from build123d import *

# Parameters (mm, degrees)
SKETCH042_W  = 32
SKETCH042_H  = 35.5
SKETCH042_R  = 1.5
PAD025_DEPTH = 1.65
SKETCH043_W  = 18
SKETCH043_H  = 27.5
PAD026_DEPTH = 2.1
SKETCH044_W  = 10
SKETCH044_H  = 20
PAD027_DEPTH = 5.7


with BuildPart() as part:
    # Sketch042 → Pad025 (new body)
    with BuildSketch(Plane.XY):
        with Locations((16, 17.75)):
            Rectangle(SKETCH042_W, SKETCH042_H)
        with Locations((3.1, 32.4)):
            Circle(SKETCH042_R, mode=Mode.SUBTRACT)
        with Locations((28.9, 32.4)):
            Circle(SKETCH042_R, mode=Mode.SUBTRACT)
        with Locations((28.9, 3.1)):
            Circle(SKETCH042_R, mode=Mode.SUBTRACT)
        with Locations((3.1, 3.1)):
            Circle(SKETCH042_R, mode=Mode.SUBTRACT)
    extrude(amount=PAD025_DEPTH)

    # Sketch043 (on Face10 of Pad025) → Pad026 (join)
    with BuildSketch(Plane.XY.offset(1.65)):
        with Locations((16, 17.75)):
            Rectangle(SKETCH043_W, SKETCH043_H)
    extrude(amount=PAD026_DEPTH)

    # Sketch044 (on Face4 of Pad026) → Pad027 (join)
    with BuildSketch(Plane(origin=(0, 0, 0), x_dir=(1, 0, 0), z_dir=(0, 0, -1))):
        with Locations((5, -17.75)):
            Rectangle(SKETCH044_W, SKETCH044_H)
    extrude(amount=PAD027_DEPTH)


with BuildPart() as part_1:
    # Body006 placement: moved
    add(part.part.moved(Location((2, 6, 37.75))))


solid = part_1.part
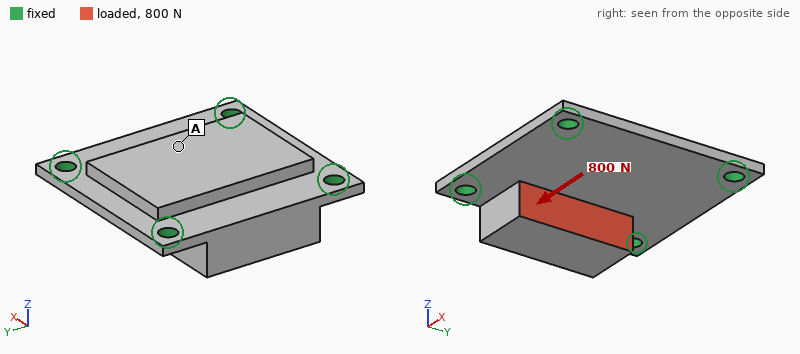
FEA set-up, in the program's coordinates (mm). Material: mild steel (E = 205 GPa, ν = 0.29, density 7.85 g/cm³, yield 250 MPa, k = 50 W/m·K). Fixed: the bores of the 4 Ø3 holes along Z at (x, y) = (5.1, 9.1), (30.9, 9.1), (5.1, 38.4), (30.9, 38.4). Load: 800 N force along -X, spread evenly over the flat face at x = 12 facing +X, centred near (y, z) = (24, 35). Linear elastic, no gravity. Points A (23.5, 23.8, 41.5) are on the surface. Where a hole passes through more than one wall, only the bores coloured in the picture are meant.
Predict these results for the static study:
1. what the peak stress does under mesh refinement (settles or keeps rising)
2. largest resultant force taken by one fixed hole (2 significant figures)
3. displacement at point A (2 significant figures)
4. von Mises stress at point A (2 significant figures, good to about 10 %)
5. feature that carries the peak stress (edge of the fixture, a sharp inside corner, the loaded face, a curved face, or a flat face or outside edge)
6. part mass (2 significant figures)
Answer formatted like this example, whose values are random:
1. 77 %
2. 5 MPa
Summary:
1. keeps rising
2. 350 N
3. 3.6 µm
4. 12 MPa
5. edge of the fixture
6. 31 g
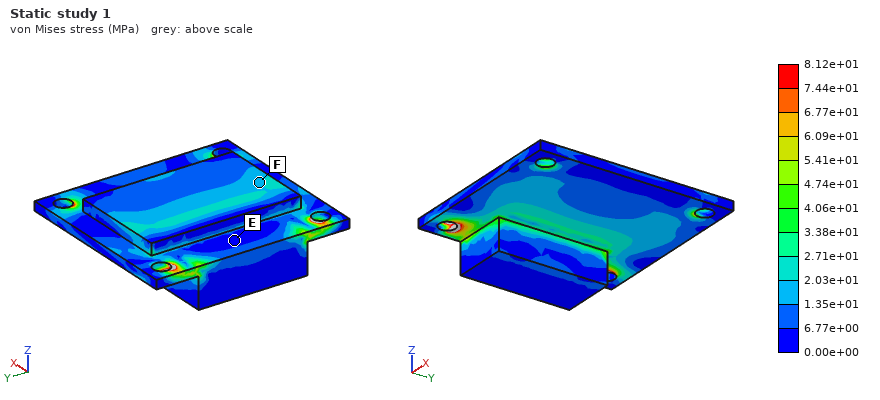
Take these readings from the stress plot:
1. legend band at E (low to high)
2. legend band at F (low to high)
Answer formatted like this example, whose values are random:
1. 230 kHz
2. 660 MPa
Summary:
1. 0.00e+00 to 6.77e+00 MPa
2. 1.35e+01 to 2.03e+01 MPa
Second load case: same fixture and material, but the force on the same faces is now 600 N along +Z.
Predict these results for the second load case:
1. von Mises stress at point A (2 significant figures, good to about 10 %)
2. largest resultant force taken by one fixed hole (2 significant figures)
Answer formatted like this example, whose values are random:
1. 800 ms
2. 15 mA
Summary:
1. 14 MPa
2. 250 N
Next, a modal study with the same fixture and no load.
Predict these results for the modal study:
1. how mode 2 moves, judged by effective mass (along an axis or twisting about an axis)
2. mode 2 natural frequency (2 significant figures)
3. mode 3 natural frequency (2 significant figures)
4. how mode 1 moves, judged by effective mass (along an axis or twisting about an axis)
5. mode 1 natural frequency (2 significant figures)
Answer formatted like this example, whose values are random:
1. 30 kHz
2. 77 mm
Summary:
1. along Z
2. 16 kHz
3. 19 kHz
4. along Z
5. 11 kHz
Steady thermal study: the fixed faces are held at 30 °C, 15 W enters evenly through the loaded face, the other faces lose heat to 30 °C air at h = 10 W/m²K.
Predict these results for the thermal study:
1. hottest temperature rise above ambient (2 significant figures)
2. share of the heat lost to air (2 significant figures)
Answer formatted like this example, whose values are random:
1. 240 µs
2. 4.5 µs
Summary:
1. 46 K
2. 3.9 %
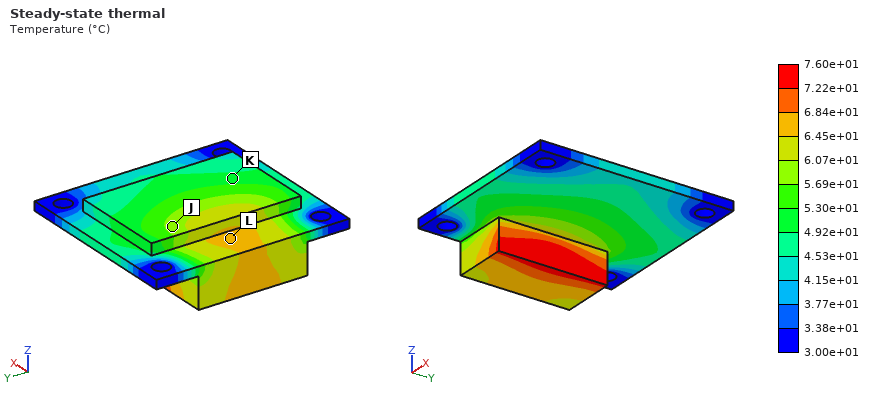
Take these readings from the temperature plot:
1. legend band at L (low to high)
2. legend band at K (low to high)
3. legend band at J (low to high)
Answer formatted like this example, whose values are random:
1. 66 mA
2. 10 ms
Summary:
1. 6.45e+01 to 6.84e+01 °C
2. 4.92e+01 to 5.30e+01 °C
3. 5.69e+01 to 6.07e+01 °C
